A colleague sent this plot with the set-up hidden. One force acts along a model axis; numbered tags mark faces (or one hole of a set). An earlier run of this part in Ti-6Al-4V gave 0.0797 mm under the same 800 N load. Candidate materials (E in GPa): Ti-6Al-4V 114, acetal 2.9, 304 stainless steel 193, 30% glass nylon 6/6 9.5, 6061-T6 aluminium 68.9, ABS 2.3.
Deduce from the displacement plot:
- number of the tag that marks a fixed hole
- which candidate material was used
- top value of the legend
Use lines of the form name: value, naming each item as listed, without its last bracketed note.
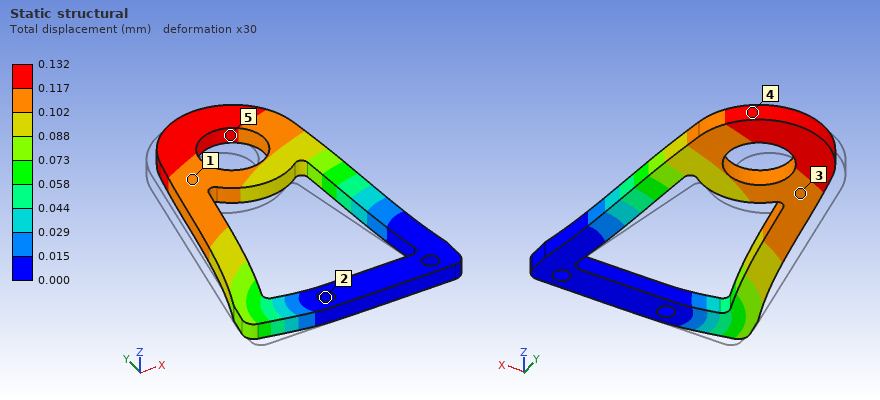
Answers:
number of the tag that marks a fixed hole: 2
which candidate material was used: 6061-T6 aluminium
top value of the legend: 0.132 mm
